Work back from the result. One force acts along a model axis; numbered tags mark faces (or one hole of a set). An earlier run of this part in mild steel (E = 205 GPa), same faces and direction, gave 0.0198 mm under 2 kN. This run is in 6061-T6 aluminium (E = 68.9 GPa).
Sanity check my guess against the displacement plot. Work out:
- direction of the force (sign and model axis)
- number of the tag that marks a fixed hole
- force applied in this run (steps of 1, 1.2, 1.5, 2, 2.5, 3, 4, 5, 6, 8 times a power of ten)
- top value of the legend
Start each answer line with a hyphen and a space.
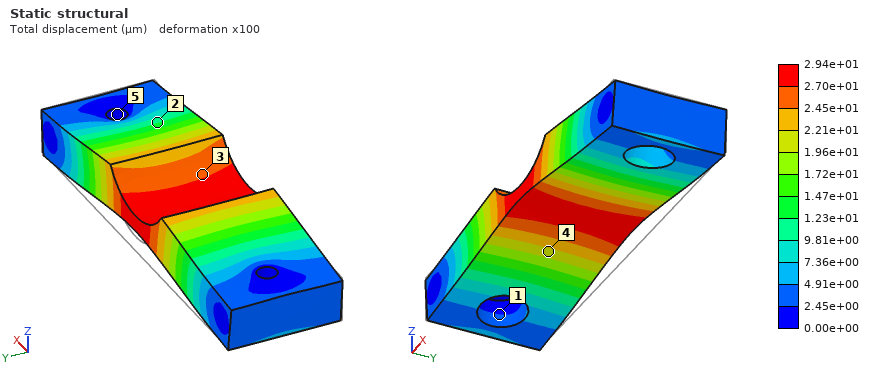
- +Z
- 5
- 1 kN
- 2.94e+01 µm
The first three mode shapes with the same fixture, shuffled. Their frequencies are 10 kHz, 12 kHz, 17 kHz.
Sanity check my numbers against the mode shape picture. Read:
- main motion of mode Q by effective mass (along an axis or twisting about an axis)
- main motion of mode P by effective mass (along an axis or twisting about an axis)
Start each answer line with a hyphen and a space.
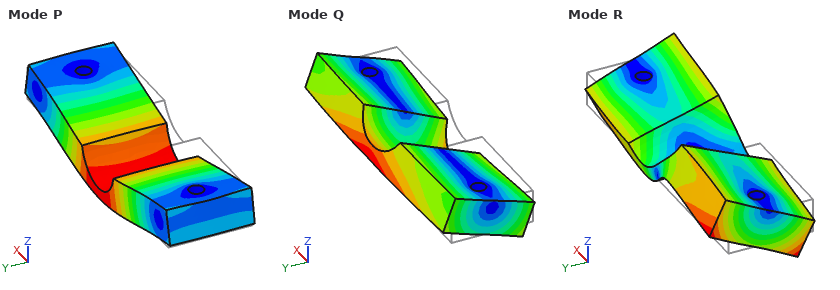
- along Y
- along Z
